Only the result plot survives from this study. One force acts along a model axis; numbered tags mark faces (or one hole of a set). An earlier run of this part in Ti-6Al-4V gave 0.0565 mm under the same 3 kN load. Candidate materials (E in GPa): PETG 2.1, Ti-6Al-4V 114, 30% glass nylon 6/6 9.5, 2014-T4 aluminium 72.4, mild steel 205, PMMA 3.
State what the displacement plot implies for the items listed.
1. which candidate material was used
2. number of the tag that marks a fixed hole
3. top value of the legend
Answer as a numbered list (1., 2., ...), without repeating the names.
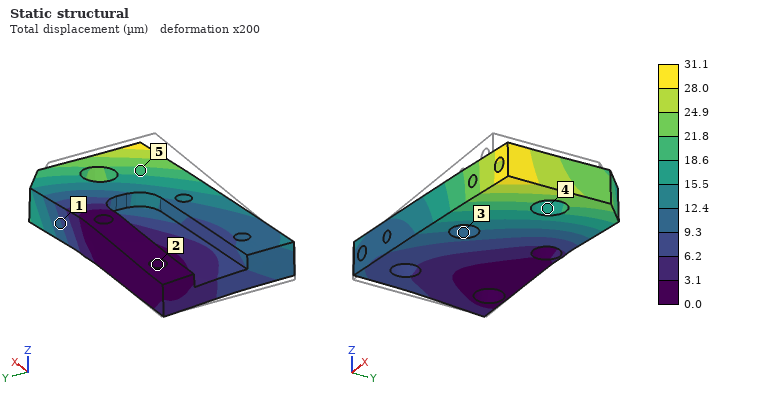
1. mild steel
2. 2
3. 31.1 µm
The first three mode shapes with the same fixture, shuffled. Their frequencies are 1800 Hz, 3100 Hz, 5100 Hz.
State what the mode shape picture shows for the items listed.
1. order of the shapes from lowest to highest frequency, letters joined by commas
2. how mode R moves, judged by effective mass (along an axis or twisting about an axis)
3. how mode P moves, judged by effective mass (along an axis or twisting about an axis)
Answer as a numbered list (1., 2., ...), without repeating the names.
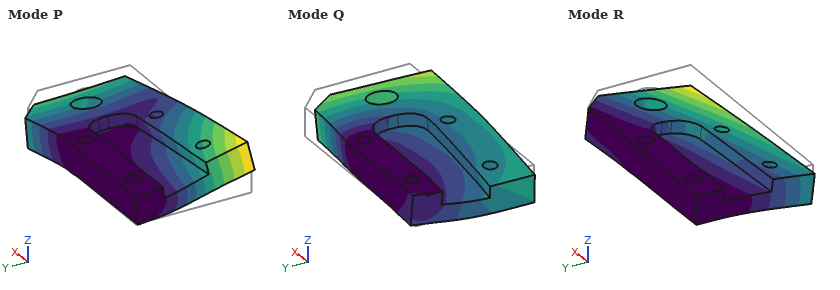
1. R, P, Q
2. along Z
3. twisting about Y
